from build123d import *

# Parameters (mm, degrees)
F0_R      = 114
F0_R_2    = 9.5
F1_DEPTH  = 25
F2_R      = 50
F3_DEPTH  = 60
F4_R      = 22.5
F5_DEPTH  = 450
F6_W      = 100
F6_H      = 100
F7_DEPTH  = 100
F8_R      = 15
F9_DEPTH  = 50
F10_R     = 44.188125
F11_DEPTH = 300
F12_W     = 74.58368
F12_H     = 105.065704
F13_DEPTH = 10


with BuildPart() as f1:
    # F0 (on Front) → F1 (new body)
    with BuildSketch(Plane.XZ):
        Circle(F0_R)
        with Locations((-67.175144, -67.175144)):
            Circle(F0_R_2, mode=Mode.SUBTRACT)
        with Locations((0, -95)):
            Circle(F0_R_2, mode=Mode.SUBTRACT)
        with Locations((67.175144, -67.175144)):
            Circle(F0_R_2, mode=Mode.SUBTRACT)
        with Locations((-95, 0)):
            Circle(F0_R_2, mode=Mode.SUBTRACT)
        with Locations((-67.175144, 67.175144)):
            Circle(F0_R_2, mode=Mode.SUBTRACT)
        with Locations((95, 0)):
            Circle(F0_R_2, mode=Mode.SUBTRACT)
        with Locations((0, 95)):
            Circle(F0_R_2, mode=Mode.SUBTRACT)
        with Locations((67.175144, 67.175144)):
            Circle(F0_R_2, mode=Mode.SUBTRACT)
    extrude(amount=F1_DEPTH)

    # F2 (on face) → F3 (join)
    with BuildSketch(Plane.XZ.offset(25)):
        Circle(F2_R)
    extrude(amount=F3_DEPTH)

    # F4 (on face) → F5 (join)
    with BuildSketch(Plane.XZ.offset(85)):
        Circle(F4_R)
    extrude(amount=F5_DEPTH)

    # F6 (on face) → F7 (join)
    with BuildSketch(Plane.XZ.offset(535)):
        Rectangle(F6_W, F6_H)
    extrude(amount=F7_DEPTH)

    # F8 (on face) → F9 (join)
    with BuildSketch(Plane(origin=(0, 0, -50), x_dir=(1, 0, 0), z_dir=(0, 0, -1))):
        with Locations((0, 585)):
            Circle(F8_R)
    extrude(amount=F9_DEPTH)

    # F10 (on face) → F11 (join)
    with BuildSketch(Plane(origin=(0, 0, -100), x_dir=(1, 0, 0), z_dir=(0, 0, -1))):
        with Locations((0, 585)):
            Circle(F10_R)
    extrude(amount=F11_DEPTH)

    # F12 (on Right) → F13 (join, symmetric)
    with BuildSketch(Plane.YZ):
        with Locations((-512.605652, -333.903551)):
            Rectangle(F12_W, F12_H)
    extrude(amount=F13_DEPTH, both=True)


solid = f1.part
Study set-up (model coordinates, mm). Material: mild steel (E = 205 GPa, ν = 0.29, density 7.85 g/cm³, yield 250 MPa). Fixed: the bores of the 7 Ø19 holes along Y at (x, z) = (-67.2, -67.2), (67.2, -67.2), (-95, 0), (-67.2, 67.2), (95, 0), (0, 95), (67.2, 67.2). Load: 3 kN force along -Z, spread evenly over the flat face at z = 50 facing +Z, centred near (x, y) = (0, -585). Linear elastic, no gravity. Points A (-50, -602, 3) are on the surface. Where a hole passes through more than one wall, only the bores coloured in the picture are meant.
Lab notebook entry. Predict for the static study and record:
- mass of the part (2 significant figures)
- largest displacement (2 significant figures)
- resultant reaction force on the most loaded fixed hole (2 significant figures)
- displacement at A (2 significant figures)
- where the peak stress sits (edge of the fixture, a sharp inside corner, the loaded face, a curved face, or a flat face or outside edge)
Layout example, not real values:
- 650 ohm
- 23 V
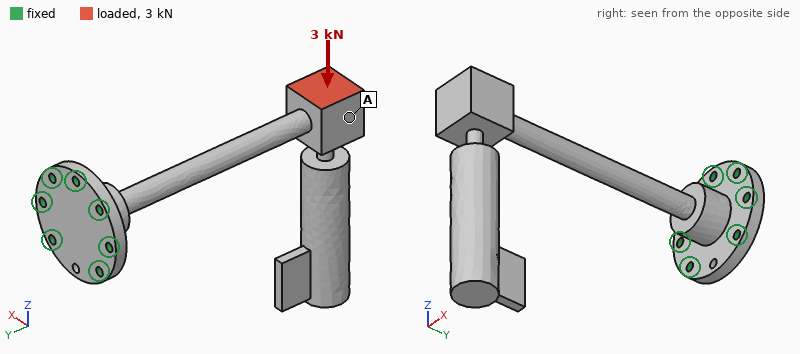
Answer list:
- 41 kg
- 5.3 mm
- 6.9 kN
- 3.5 mm
- a curved face
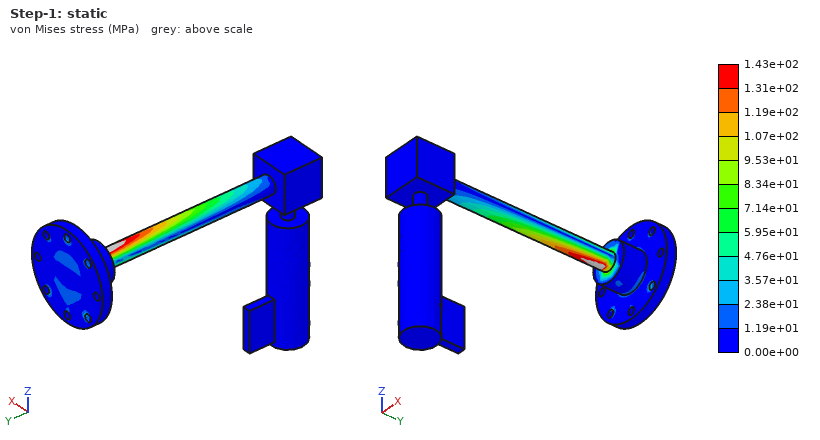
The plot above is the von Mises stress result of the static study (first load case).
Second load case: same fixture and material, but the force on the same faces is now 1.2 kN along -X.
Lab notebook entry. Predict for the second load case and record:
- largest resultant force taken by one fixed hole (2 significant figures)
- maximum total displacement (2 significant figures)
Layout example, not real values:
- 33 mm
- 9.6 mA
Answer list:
- 2.3 kN
- 1.6 mm
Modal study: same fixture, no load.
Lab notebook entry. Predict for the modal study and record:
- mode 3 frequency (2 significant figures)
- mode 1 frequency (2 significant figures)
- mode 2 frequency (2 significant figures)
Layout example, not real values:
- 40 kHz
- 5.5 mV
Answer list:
- 63 Hz
- 25 Hz
- 25 Hz
